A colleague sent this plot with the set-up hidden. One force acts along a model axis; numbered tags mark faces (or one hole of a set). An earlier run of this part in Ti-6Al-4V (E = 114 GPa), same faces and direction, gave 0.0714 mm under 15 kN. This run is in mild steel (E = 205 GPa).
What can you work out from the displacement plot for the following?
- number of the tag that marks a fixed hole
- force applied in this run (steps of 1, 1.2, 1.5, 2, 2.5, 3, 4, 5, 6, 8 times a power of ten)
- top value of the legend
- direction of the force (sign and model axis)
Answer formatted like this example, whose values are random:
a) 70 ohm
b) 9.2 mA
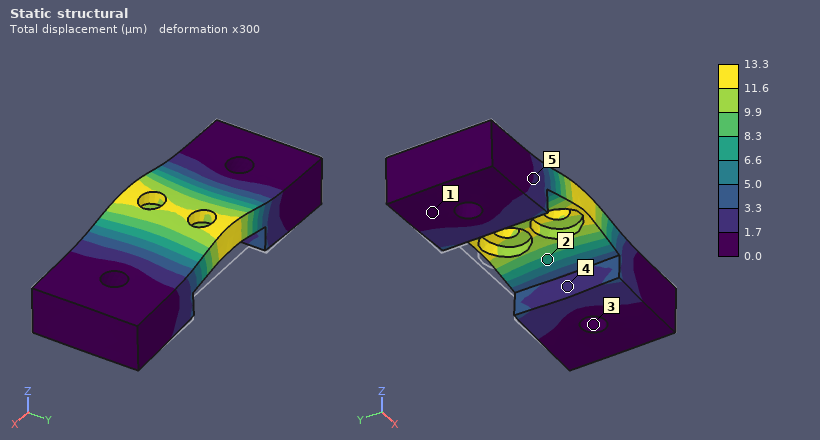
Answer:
a) 3
b) 5 kN
c) 13.3 µm
d) +Z
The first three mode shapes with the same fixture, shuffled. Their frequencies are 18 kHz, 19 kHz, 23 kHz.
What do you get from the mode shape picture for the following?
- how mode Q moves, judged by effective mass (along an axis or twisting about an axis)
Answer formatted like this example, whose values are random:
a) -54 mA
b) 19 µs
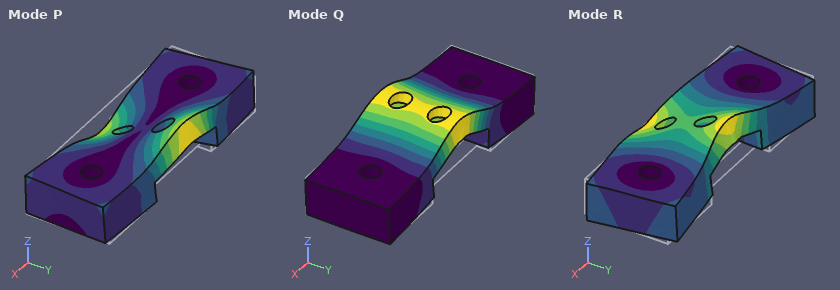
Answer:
a) along Z
